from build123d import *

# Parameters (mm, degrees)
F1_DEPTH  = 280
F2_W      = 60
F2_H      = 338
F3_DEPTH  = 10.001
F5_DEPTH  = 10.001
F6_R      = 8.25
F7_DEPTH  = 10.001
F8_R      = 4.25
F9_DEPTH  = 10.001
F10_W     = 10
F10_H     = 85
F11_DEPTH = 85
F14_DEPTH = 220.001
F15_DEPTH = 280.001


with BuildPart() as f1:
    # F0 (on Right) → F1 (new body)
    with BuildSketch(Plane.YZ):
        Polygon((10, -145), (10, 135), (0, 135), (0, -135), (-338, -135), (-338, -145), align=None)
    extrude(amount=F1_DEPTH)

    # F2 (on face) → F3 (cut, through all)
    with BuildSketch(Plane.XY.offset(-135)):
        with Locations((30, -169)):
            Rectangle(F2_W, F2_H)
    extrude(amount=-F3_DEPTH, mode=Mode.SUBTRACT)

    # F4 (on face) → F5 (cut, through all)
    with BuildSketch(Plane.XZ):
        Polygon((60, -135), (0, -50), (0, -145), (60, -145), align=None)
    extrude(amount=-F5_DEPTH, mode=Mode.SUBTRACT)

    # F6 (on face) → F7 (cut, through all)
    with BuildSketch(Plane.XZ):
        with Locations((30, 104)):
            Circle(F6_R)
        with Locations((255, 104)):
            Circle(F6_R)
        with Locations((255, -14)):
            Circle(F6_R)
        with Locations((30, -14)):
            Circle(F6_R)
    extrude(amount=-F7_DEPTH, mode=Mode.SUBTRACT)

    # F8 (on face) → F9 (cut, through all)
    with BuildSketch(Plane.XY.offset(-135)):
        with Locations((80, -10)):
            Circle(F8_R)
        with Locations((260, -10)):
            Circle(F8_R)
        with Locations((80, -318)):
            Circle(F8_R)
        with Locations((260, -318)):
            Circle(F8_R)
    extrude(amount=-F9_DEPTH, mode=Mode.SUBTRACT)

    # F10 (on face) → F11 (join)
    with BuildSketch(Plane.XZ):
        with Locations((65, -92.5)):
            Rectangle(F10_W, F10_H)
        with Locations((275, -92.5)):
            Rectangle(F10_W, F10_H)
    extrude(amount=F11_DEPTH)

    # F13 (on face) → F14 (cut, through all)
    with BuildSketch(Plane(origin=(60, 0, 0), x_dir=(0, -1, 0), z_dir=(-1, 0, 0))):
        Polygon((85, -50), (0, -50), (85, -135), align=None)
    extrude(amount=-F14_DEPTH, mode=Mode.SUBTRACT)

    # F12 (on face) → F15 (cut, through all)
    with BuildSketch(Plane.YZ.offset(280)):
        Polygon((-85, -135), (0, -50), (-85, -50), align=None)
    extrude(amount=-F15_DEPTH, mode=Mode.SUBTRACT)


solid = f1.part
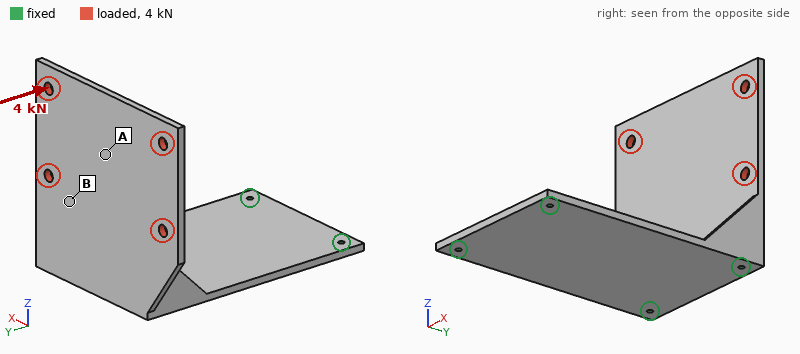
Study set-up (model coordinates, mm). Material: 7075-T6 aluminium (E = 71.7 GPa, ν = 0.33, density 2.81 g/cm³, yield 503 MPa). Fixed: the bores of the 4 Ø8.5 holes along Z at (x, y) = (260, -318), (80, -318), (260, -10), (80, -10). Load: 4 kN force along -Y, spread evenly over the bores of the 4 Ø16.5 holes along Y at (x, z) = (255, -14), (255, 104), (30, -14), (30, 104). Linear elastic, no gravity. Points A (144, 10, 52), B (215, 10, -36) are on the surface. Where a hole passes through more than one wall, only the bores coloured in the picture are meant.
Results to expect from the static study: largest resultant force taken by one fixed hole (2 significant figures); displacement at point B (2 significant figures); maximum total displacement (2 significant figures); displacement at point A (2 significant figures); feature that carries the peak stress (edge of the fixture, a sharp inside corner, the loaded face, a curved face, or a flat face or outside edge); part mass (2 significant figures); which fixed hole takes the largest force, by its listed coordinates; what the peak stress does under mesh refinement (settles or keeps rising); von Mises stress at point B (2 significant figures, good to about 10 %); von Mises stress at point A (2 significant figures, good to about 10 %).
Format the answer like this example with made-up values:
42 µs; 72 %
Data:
2.0 kN; 1.1 mm; 5.8 mm; 3.2 mm; edge of the fixture; 4.4 kg; (80, -10); keeps rising; 62 MPa; 22 MPa
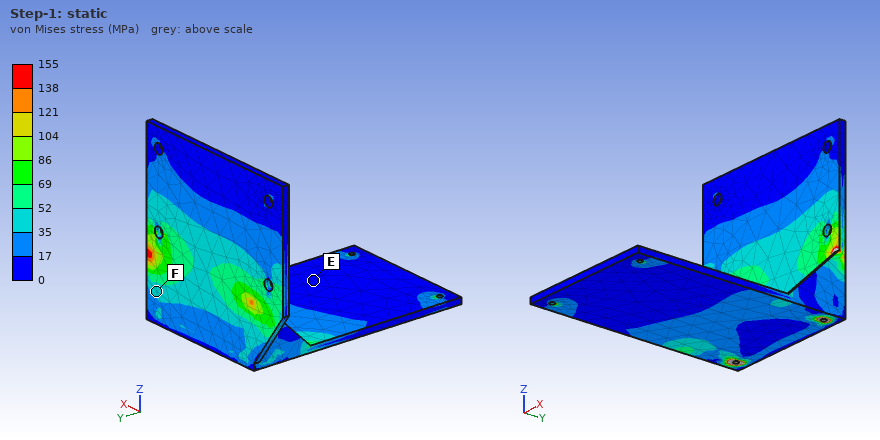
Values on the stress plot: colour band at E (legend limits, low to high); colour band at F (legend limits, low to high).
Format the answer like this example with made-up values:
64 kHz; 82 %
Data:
0 to 17 MPa; 35 to 52 MPa
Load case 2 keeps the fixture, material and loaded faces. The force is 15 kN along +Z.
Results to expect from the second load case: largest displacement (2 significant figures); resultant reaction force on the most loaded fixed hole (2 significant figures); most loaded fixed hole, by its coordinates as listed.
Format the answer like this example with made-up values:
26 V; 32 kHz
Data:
0.62 mm; 9.8 kN; (80, -10)
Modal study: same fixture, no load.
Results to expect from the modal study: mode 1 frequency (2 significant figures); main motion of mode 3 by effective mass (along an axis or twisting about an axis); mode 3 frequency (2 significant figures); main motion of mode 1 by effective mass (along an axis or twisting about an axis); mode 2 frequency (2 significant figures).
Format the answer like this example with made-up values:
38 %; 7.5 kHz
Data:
140 Hz; along Z; 500 Hz; along Y; 300 Hz
